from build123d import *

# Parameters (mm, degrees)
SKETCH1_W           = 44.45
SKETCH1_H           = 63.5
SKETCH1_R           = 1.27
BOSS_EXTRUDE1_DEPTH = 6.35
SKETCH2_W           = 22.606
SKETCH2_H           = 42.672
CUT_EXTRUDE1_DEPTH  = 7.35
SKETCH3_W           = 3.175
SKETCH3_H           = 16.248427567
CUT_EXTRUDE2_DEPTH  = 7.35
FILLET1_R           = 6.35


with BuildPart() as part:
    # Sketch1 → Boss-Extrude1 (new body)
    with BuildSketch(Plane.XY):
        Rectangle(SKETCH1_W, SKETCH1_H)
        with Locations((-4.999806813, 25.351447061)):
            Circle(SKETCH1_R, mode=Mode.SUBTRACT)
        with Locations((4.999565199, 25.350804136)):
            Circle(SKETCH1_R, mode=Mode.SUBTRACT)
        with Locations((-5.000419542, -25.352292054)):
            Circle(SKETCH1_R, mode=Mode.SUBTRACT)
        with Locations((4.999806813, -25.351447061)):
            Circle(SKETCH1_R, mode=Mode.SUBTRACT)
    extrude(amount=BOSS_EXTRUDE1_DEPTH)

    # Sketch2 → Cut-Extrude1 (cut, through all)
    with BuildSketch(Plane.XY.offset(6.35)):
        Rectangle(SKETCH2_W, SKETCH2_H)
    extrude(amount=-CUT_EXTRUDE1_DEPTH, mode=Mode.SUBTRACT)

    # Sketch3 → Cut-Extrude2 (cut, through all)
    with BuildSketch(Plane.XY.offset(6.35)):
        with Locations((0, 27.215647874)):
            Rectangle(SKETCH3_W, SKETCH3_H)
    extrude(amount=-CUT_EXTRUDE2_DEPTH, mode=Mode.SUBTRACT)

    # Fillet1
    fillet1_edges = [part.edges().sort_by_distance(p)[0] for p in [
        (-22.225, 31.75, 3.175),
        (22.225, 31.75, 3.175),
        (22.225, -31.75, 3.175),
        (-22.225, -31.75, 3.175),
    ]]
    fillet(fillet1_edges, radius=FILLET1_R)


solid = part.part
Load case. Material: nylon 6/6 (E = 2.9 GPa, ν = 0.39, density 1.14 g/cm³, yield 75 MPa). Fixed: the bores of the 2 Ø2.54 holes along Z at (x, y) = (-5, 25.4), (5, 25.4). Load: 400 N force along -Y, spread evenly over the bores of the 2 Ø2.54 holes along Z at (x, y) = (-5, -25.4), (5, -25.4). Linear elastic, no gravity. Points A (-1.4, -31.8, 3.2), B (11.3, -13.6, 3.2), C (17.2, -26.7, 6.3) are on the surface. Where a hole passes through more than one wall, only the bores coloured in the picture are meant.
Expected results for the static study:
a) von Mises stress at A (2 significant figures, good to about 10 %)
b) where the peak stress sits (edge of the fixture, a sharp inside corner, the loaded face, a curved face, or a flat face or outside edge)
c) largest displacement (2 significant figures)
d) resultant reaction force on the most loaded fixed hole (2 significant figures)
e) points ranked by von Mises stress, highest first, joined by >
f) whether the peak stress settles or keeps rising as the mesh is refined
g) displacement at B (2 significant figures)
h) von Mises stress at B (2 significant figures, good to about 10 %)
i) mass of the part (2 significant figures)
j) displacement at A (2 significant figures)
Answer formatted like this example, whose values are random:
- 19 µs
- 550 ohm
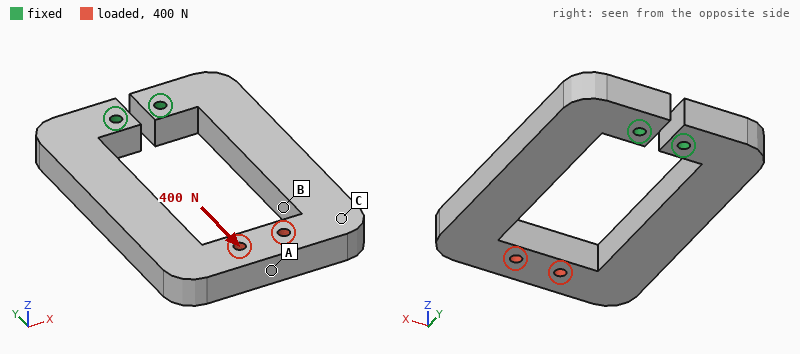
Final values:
- 16 MPa
- edge of the fixture
- 0.33 mm
- 200 N
- A > B > C
- keeps rising
- 0.24 mm
- 9.2 MPa
- 13 g
- 0.32 mm
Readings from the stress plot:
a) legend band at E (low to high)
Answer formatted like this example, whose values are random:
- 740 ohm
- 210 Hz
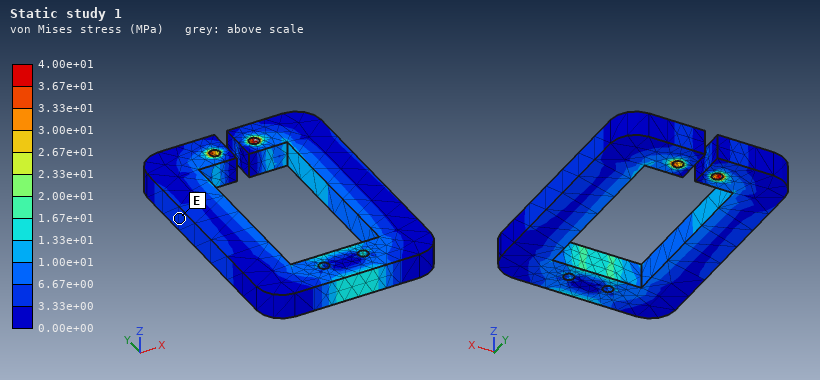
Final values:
- 3.33e+00 to 6.67e+00 MPa
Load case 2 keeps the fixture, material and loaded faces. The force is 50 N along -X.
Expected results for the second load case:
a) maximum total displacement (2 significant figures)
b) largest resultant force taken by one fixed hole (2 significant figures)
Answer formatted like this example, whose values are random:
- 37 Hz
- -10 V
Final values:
- 0.79 mm
- 50 N
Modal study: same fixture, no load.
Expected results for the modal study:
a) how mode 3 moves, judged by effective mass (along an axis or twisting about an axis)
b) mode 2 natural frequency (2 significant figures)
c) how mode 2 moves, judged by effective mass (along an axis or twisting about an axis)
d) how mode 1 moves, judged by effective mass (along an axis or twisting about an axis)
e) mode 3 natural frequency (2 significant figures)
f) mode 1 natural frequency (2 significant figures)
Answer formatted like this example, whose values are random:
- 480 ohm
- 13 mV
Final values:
- twisting about Y
- 550 Hz
- along X
- along Z
- 790 Hz
- 310 Hz
